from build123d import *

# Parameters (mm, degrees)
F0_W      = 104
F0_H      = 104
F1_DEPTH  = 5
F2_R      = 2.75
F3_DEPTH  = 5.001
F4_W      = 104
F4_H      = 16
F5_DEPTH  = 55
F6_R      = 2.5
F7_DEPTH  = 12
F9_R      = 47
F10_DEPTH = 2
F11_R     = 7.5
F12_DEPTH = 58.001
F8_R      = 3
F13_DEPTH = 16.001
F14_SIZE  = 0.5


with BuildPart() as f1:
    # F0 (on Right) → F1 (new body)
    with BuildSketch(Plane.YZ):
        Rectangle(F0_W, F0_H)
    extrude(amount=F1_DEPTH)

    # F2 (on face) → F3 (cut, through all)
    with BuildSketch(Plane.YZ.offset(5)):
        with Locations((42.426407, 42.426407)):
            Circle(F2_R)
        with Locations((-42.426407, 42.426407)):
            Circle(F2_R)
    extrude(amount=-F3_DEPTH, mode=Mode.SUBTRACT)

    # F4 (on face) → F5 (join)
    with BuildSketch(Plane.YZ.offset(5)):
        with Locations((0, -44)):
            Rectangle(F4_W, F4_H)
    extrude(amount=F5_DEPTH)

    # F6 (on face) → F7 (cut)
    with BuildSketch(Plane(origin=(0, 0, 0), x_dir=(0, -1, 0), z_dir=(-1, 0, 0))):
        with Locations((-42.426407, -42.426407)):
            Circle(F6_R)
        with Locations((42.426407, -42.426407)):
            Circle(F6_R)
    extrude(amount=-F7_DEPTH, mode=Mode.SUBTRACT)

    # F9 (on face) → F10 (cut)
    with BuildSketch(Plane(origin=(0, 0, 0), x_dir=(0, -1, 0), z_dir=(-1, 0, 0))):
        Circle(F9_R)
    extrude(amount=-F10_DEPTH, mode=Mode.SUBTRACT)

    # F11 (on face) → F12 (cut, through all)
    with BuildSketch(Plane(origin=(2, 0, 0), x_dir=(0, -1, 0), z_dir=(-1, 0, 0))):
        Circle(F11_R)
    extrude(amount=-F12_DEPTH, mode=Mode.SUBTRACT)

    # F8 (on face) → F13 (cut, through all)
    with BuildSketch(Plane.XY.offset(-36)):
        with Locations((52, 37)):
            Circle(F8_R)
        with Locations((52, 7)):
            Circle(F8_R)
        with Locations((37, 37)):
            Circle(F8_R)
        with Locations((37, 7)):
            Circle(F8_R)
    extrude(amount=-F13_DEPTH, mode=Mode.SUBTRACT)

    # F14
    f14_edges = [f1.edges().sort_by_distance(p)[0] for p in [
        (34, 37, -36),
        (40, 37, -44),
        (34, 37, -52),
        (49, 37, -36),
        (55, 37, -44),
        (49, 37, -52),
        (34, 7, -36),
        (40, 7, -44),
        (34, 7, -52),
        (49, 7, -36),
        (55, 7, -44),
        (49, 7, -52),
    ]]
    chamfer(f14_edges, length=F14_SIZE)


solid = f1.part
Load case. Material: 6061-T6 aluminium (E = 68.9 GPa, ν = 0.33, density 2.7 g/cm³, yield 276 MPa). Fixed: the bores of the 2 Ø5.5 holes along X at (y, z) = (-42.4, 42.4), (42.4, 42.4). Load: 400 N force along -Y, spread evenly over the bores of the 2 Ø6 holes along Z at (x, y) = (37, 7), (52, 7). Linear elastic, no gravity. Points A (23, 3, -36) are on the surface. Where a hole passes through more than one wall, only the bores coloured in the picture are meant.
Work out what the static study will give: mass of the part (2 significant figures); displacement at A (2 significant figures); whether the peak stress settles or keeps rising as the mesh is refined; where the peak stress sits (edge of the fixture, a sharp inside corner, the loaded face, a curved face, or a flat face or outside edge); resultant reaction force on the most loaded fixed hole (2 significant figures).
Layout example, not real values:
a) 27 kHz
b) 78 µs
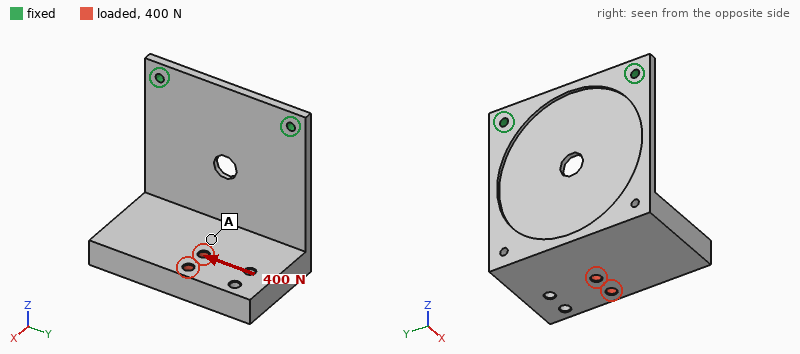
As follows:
a) 350 g
b) 0.20 mm
c) keeps rising
d) edge of the fixture
e) 480 N
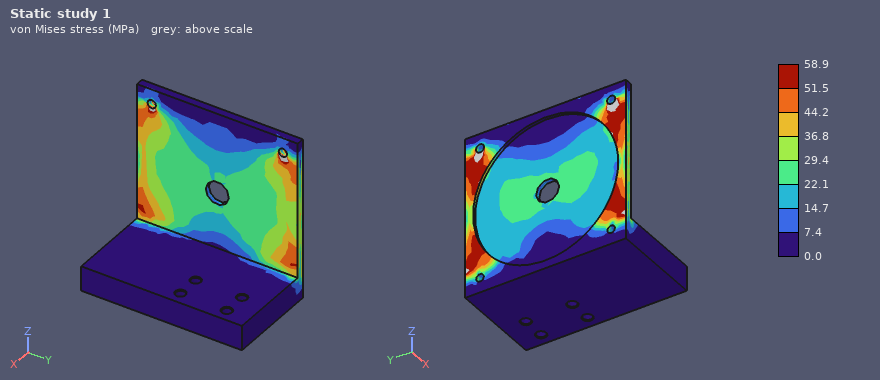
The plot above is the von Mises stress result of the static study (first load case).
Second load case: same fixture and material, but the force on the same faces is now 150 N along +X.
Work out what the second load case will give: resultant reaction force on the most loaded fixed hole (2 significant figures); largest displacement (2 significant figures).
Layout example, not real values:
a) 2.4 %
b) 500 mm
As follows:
a) 210 N
b) 1.6 mm
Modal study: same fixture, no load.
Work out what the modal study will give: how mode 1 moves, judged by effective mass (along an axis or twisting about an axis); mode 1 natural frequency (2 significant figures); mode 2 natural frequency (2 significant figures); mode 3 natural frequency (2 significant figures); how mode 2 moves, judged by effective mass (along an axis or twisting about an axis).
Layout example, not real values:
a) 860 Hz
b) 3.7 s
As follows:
a) along X
b) 100 Hz
c) 280 Hz
d) 480 Hz
e) along Y
